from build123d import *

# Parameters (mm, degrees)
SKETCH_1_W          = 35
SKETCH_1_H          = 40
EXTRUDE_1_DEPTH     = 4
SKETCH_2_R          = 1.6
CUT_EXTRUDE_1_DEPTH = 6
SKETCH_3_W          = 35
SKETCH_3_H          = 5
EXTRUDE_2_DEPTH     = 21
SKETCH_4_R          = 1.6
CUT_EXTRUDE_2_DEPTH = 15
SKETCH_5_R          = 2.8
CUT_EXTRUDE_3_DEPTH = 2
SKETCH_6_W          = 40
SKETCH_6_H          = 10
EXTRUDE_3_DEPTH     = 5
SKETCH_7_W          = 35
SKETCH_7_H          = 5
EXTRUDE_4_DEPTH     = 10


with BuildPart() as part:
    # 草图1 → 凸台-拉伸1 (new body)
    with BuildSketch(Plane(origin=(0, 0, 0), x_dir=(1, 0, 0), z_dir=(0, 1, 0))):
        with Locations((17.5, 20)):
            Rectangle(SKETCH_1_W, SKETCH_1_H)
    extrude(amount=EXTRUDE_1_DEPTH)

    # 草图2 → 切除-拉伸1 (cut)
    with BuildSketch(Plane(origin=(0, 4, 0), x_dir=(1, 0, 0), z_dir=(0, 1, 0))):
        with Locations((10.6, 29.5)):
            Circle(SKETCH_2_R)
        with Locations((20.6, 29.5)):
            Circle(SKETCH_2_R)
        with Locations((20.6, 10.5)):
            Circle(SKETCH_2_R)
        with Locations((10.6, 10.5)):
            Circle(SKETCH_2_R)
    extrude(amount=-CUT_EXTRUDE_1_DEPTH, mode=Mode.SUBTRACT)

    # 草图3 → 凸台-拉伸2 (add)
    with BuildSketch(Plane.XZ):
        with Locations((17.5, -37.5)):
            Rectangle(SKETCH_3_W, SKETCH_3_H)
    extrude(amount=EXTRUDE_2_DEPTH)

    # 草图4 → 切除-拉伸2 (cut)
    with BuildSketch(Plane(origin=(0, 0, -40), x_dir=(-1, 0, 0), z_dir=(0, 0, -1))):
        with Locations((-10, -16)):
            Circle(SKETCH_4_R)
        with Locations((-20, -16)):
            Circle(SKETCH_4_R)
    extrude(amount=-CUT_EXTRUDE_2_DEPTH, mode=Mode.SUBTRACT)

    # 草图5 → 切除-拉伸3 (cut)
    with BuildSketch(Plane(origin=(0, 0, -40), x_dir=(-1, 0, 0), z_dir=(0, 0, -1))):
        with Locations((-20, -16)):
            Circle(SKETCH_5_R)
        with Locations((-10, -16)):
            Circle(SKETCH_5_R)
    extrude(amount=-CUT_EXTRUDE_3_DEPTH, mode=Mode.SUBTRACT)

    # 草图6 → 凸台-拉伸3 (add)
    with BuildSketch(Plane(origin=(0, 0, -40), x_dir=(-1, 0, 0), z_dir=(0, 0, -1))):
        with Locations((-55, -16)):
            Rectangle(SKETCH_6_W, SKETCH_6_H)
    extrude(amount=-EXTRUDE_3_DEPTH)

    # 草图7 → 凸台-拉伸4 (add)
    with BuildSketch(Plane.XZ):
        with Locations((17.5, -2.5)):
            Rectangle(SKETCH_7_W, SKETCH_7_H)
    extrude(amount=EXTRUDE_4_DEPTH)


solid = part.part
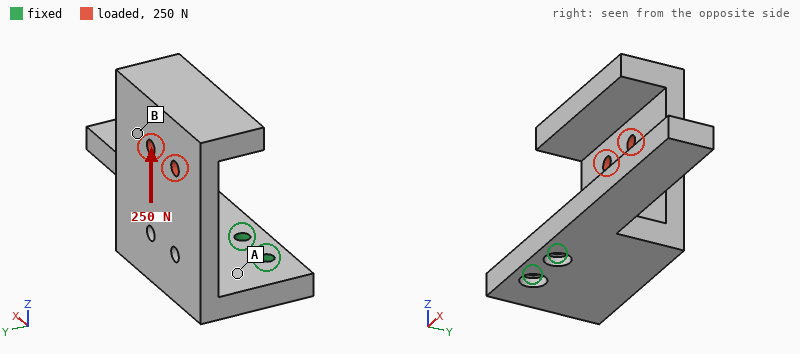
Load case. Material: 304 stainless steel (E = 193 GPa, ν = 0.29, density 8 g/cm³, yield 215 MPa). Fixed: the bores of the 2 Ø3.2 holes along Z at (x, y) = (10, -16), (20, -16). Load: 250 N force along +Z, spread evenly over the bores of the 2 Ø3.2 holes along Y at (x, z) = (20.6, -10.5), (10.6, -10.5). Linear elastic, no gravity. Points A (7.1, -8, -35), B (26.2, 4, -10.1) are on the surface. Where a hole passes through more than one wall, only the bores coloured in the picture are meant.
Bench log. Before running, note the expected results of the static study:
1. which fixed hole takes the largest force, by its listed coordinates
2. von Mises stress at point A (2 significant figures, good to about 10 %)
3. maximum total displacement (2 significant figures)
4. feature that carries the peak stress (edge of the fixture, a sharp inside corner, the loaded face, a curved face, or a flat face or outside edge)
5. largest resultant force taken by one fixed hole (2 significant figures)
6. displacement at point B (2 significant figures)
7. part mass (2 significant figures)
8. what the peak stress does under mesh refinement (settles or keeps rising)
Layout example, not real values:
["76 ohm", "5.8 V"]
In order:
["(20, -16)", "17 MPa", "42 µm", "edge of the fixture", "140 N", "33 µm", "100 g", "keeps rising"]
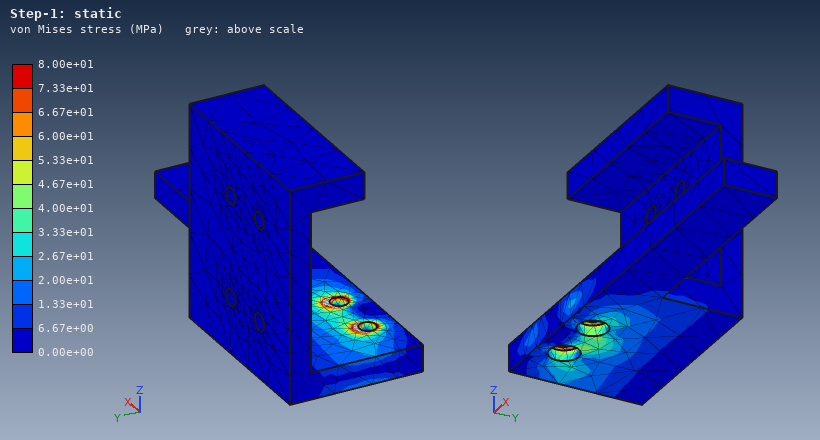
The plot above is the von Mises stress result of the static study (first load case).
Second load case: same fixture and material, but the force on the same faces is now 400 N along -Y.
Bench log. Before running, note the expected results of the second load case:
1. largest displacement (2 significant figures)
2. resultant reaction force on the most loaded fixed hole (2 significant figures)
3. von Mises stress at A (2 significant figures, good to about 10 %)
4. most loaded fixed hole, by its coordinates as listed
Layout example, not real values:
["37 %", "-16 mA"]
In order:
["0.26 mm", "270 N", "76 MPa", "(20, -16)"]
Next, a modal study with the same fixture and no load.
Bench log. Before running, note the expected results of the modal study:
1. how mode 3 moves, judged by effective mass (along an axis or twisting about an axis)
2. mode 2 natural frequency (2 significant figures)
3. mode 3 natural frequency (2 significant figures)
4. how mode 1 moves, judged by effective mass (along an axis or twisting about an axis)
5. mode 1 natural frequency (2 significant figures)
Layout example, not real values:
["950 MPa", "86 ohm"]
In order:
["along X", "1400 Hz", "1900 Hz", "along Y", "1000 Hz"]
